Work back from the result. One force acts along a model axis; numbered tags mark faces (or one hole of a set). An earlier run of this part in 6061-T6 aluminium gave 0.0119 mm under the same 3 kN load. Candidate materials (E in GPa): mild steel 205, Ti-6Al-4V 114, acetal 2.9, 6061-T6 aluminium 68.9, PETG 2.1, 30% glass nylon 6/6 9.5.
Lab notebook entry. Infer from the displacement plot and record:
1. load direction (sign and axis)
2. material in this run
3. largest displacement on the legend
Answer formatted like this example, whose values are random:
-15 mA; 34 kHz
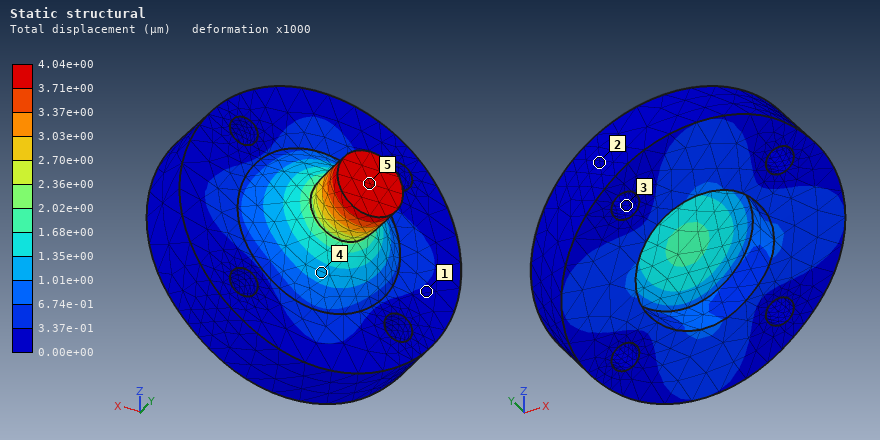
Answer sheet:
-Y; mild steel; 4.04e+00 µm
